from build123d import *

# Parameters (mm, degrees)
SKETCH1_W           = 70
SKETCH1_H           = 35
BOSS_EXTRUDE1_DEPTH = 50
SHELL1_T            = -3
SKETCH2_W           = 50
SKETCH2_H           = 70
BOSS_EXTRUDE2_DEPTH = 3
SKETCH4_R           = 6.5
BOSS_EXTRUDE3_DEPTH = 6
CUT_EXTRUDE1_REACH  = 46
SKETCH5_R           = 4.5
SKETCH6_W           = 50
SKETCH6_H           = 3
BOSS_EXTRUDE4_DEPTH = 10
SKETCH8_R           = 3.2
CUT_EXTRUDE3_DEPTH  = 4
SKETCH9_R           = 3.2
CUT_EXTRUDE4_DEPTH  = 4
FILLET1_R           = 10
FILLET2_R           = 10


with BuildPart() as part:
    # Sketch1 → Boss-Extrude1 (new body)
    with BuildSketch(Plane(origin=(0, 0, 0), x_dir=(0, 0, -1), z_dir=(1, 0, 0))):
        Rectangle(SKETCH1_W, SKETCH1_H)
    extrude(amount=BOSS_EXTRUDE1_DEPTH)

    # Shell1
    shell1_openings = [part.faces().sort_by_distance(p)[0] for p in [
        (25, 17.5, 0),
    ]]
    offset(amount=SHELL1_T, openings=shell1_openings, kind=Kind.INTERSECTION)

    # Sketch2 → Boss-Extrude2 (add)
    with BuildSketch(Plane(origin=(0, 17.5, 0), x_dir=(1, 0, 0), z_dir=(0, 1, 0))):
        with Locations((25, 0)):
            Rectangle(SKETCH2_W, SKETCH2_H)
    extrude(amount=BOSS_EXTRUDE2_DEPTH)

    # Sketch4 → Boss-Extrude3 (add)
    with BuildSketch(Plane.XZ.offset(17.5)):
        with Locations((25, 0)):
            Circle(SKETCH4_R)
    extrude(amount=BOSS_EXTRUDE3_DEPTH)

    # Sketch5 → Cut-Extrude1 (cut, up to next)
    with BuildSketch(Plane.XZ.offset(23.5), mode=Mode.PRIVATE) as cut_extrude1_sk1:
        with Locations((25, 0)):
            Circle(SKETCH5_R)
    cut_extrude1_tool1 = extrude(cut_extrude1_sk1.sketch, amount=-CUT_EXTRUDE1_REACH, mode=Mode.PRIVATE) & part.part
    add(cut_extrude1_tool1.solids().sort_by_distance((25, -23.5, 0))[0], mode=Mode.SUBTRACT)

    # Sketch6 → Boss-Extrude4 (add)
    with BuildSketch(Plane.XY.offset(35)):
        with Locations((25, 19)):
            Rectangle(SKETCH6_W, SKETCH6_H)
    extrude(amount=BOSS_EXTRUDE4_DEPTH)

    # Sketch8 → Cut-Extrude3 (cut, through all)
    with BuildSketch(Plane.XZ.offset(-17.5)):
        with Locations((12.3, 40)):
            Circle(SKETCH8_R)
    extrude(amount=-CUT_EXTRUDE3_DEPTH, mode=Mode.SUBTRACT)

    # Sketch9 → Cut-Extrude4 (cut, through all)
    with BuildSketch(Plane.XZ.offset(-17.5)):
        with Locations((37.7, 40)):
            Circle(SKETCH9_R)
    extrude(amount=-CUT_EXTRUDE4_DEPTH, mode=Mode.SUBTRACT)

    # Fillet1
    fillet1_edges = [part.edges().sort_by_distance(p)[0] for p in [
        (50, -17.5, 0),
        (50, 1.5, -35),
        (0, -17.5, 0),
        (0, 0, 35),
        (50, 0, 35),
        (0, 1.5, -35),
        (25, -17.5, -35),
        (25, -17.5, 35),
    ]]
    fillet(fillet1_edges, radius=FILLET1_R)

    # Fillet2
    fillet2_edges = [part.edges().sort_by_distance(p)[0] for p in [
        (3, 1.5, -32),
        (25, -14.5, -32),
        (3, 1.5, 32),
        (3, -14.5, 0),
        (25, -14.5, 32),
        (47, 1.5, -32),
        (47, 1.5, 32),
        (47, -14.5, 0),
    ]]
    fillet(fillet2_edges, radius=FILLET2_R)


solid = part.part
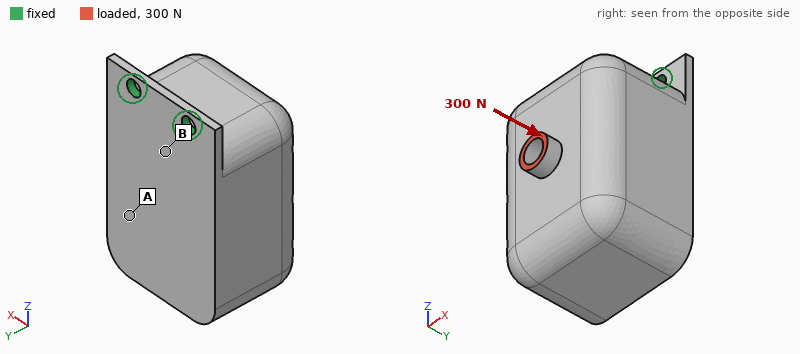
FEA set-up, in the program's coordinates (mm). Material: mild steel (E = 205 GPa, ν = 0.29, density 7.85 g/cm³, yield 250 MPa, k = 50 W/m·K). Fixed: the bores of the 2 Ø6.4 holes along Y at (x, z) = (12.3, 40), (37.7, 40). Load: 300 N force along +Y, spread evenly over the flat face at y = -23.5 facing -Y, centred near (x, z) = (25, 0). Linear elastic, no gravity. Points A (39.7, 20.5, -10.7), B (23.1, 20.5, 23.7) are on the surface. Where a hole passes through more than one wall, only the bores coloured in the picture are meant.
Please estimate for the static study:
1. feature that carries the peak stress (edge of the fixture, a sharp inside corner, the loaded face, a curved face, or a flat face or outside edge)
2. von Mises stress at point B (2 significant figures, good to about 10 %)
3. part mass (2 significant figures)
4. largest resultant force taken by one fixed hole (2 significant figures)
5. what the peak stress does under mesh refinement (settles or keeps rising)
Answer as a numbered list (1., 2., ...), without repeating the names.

1. edge of the fixture
2. 22 MPa
3. 340 g
4. 160 N
5. keeps rising
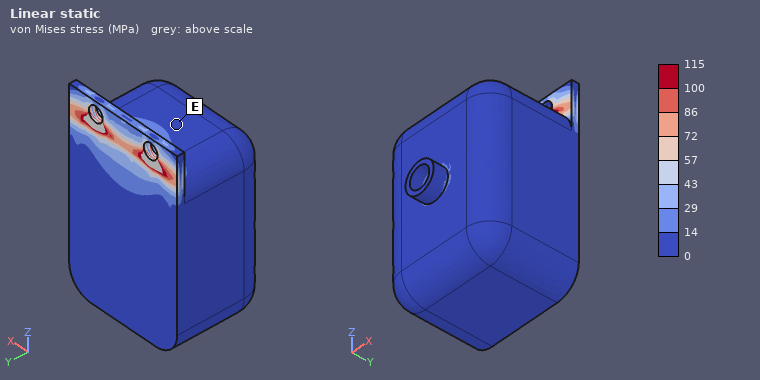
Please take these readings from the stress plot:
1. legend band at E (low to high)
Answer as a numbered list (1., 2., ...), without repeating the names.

1. 0 to 14 MPa
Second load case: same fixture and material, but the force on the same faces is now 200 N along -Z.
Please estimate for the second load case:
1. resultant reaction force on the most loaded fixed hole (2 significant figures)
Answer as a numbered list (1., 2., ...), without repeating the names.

1. 100 N
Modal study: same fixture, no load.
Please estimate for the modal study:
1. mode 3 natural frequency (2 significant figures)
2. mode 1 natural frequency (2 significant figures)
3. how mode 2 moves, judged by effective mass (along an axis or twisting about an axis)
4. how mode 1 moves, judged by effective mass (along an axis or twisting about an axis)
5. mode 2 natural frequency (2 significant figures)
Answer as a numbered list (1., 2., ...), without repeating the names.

1. 3400 Hz
2. 340 Hz
3. along X
4. along Y
5. 2300 Hz
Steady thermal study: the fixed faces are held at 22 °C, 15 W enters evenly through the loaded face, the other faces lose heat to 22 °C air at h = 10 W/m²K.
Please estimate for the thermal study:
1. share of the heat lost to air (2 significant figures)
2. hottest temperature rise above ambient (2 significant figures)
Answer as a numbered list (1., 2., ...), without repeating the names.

1. 42 %
2. 80 K
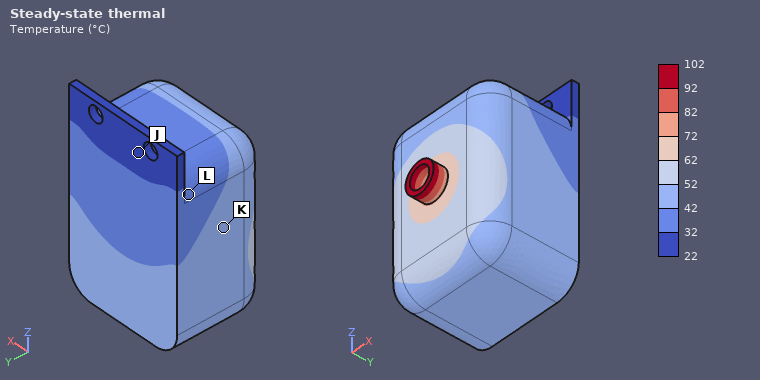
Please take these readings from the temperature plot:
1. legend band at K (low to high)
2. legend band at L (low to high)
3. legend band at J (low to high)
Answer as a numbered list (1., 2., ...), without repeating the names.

1. 42 to 52 °C
2. 32 to 42 °C
3. 22 to 32 °C
